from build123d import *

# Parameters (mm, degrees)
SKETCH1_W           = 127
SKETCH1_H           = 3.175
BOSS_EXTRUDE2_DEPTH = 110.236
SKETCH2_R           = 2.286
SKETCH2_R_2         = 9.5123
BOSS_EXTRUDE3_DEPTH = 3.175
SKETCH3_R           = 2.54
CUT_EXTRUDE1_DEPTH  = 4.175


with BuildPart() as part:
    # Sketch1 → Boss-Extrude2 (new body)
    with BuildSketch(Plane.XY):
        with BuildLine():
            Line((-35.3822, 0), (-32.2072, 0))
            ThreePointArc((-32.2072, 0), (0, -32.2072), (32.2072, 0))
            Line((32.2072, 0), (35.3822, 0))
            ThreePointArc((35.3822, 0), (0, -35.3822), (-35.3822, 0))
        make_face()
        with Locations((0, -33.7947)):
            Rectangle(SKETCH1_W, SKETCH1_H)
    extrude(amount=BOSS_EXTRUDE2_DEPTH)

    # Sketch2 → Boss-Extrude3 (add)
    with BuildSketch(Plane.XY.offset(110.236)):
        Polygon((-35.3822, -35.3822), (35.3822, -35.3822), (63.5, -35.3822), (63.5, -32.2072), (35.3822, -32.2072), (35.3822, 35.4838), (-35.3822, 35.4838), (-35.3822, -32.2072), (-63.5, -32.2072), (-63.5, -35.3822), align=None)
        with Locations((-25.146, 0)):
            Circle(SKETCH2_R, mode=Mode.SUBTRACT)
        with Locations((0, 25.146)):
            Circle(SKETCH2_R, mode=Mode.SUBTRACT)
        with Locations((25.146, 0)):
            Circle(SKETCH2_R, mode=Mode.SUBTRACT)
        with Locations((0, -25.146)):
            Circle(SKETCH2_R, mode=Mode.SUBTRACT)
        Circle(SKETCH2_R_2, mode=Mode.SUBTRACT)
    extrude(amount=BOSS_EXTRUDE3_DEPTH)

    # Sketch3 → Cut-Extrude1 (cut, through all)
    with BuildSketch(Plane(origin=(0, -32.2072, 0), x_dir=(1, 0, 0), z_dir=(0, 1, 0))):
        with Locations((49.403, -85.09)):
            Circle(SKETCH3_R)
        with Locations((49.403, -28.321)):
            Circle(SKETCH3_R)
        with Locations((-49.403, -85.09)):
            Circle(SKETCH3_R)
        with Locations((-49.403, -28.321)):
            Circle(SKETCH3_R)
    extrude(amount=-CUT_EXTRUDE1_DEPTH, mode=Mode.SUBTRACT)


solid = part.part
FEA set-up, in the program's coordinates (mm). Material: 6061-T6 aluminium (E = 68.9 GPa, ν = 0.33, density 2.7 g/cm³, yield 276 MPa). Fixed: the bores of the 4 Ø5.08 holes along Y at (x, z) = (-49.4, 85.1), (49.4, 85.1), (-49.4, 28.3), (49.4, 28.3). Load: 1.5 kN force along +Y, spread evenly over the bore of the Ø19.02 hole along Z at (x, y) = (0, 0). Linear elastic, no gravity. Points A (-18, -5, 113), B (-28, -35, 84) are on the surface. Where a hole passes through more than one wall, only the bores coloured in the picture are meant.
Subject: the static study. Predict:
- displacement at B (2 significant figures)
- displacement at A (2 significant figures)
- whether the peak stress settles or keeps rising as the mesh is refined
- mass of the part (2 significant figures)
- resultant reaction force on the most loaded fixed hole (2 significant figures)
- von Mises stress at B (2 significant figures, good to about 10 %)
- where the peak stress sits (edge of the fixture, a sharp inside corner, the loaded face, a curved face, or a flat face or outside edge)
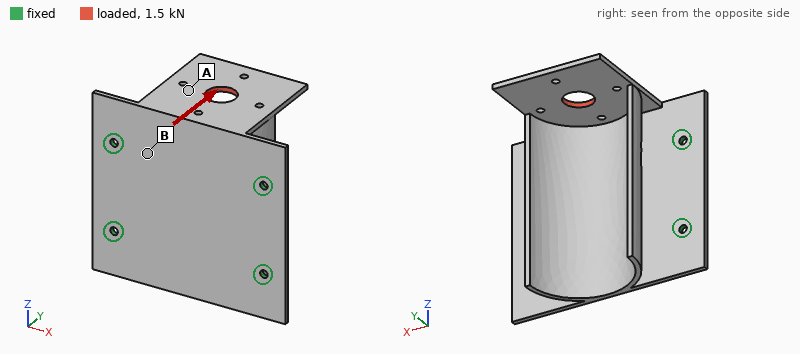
0.19 mm
0.53 mm
keeps rising
240 g
1.0 kN
51 MPa
edge of the fixture
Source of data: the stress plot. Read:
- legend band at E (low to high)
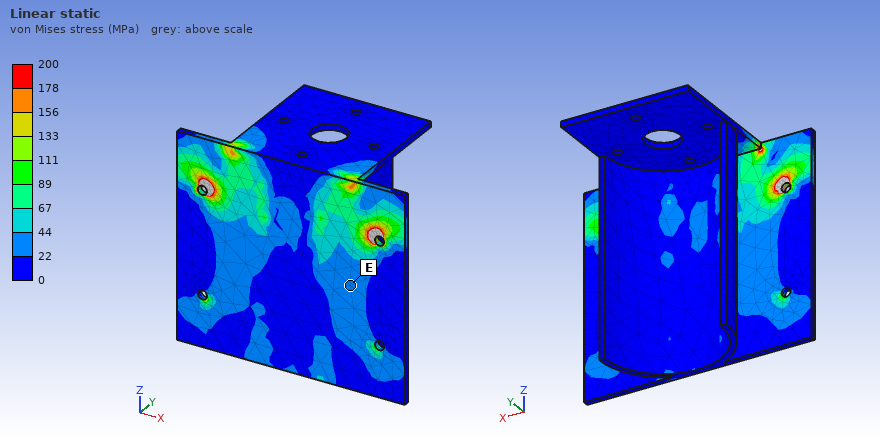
22 to 44 MPa
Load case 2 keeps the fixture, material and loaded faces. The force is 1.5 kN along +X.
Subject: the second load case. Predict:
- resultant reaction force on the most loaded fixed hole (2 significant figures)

990 N
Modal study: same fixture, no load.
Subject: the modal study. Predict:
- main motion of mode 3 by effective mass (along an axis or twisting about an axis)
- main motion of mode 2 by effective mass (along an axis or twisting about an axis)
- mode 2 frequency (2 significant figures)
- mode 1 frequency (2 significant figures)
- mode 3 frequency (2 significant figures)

along X
along Y
1100 Hz
800 Hz
1200 Hz
